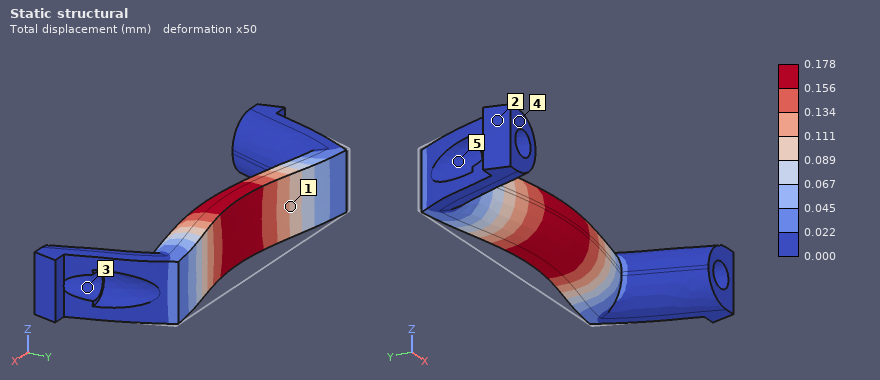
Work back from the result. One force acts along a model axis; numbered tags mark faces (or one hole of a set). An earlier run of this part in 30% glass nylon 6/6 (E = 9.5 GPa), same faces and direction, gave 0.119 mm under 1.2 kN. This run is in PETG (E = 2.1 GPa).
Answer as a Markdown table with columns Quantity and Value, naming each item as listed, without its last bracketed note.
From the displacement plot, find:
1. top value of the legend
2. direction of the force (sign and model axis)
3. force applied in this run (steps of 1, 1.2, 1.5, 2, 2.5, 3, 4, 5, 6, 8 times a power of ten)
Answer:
| Quantity | Value |
|---|---|
| top value of the legend | 0.178 mm |
| direction of the force | -Y |
| force applied in this run | 400 N |
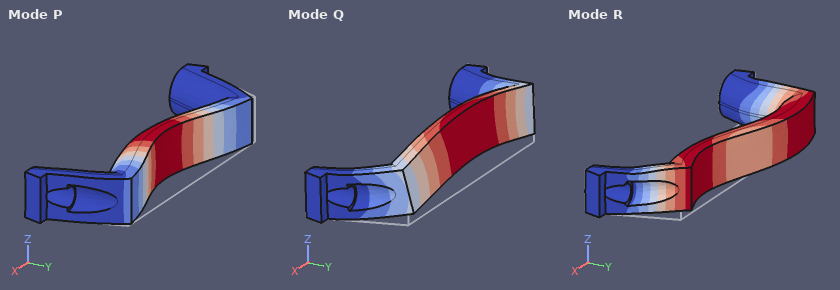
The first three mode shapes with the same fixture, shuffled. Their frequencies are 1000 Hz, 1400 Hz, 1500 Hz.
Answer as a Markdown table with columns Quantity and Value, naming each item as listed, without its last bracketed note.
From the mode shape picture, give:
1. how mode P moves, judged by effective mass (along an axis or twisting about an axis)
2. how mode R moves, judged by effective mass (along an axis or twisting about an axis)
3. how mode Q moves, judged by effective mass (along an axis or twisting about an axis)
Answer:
| Quantity | Value |
|---|---|
| how mode P moves, judged by effective mass | along Y |
| how mode R moves, judged by effective mass | along X |
| how mode Q moves, judged by effective mass | along Z |
